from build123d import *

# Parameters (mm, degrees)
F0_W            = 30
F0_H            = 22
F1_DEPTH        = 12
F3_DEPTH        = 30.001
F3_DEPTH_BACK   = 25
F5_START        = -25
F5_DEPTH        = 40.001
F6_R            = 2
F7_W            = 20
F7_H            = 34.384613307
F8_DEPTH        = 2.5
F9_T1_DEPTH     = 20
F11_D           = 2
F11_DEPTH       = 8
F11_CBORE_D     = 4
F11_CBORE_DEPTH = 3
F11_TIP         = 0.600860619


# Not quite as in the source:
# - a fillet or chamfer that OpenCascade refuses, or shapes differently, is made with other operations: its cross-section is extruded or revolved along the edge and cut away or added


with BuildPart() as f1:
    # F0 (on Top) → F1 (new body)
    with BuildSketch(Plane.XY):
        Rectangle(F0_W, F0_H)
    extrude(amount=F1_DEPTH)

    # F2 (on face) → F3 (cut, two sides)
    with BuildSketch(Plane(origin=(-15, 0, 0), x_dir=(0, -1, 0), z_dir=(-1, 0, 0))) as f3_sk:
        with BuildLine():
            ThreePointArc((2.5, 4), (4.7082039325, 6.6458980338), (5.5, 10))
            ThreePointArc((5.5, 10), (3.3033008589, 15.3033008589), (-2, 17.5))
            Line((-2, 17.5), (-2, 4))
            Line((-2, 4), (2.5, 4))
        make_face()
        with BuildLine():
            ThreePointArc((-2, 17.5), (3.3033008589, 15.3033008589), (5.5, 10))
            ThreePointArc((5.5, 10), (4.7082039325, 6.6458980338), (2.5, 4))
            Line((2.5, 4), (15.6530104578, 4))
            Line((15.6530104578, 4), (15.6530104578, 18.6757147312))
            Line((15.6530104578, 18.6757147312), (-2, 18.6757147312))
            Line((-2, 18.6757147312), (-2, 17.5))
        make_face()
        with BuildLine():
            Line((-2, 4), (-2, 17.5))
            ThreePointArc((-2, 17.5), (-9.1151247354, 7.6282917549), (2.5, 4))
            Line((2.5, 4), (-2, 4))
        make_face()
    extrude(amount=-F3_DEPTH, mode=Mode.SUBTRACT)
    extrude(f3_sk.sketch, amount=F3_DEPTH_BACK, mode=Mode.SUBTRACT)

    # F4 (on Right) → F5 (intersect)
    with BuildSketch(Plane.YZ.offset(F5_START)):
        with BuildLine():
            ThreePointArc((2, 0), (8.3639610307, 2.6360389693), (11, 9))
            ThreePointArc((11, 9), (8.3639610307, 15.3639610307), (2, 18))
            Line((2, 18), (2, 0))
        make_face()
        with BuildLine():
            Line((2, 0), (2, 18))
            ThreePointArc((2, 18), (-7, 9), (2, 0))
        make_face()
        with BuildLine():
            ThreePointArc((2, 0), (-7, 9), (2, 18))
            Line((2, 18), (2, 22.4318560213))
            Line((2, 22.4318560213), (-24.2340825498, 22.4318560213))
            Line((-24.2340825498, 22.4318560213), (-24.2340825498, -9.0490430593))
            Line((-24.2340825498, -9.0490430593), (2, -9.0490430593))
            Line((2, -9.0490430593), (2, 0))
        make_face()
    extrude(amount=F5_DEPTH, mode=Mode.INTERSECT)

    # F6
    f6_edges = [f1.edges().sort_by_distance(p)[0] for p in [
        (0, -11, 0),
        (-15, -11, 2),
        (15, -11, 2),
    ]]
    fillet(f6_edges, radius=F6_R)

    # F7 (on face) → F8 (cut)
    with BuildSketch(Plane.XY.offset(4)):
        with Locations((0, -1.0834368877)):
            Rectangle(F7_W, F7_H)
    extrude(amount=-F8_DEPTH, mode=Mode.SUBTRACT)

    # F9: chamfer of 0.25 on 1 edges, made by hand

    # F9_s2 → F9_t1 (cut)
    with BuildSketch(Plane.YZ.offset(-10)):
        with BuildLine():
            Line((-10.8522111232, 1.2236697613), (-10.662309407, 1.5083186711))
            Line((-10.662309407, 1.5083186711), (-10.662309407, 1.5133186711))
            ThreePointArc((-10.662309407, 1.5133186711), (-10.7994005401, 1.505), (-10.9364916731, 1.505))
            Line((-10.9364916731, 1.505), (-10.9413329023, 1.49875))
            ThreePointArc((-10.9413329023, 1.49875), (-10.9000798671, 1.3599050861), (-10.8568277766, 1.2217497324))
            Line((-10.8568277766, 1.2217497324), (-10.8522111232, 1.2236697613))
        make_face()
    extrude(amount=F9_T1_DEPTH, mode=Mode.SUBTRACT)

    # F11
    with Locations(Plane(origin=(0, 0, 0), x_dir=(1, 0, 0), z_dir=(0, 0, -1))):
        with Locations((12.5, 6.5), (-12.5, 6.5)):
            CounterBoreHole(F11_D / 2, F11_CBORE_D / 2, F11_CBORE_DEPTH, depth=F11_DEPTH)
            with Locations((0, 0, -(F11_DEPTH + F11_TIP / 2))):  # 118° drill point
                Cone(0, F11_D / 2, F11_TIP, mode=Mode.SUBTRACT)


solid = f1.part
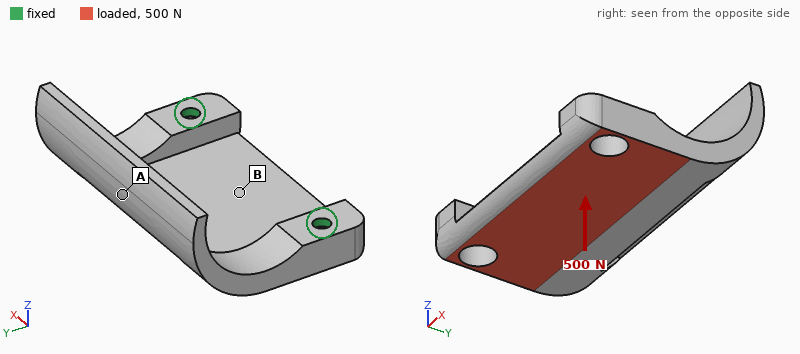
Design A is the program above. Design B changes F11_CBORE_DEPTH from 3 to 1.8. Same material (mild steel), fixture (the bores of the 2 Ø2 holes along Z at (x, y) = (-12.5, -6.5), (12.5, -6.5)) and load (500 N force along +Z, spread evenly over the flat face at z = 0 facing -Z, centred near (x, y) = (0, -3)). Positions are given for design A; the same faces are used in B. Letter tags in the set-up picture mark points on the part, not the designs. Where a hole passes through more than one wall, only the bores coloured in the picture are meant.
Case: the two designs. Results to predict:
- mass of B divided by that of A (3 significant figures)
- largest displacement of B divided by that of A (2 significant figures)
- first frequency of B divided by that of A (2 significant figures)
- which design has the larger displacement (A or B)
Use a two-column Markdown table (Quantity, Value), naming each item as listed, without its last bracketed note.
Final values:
| Quantity | Value |
|---|---|
| mass of B divided by that of A | 1.02 |
| largest displacement of B divided by that of A | 0.49 |
| first frequency of B divided by that of A | 1.3 |
| which design has the larger displacement | A |
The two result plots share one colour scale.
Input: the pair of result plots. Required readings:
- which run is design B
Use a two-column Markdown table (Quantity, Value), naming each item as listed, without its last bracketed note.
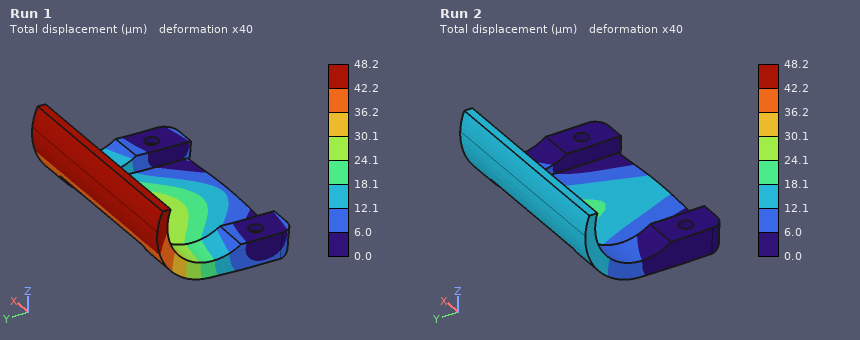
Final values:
| Quantity | Value |
|---|---|
| which run is design B | Run 2 |
